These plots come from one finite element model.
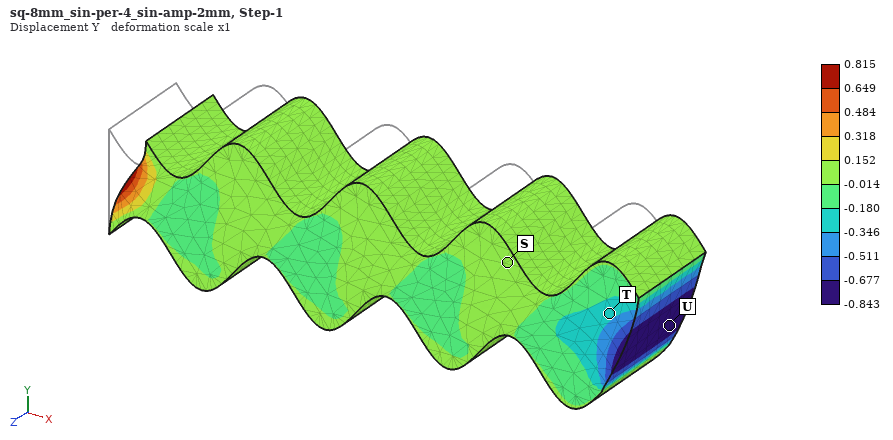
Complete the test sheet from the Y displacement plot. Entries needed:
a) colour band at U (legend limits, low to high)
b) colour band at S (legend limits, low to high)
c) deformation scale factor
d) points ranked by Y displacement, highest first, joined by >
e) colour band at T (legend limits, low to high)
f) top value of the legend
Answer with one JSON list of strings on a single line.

["-0.843 to -0.677", "-0.014 to 0.152", "1", "S > T > U", "-0.346 to -0.180", "0.815"]
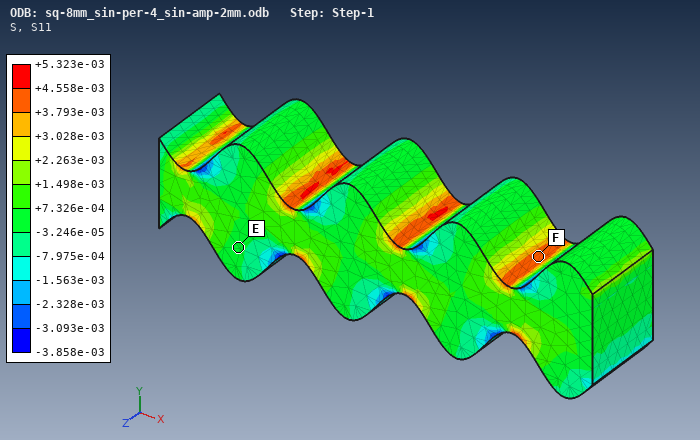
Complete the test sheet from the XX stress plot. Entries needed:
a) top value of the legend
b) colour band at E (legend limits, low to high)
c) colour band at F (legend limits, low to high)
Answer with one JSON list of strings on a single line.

["+5.323e-03", "-3.246e-05 to +7.326e-04", "+3.793e-03 to +4.558e-03"]
